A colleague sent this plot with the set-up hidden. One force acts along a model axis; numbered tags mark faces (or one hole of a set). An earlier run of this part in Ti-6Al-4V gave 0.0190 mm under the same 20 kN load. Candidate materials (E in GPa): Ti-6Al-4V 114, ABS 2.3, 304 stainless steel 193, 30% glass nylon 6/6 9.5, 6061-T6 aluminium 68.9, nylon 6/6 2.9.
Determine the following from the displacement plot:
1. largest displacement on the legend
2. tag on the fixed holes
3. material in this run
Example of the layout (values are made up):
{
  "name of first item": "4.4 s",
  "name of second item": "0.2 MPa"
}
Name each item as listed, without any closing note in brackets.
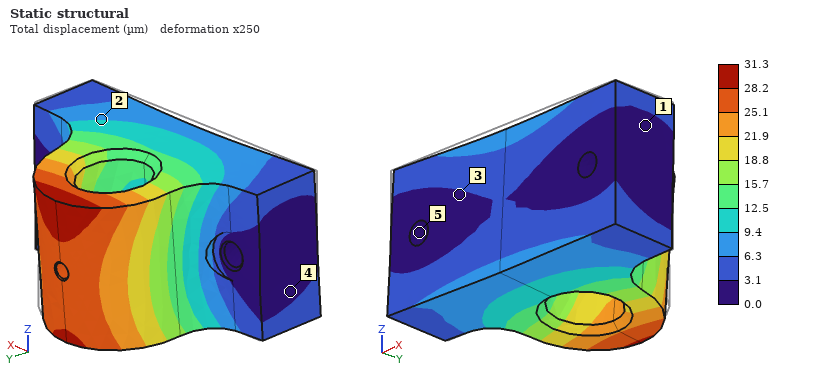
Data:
{
  "largest displacement on the legend": "31.3 µm",
  "tag on the fixed holes": "5",
  "material in this run": "6061-T6 aluminium"
}
